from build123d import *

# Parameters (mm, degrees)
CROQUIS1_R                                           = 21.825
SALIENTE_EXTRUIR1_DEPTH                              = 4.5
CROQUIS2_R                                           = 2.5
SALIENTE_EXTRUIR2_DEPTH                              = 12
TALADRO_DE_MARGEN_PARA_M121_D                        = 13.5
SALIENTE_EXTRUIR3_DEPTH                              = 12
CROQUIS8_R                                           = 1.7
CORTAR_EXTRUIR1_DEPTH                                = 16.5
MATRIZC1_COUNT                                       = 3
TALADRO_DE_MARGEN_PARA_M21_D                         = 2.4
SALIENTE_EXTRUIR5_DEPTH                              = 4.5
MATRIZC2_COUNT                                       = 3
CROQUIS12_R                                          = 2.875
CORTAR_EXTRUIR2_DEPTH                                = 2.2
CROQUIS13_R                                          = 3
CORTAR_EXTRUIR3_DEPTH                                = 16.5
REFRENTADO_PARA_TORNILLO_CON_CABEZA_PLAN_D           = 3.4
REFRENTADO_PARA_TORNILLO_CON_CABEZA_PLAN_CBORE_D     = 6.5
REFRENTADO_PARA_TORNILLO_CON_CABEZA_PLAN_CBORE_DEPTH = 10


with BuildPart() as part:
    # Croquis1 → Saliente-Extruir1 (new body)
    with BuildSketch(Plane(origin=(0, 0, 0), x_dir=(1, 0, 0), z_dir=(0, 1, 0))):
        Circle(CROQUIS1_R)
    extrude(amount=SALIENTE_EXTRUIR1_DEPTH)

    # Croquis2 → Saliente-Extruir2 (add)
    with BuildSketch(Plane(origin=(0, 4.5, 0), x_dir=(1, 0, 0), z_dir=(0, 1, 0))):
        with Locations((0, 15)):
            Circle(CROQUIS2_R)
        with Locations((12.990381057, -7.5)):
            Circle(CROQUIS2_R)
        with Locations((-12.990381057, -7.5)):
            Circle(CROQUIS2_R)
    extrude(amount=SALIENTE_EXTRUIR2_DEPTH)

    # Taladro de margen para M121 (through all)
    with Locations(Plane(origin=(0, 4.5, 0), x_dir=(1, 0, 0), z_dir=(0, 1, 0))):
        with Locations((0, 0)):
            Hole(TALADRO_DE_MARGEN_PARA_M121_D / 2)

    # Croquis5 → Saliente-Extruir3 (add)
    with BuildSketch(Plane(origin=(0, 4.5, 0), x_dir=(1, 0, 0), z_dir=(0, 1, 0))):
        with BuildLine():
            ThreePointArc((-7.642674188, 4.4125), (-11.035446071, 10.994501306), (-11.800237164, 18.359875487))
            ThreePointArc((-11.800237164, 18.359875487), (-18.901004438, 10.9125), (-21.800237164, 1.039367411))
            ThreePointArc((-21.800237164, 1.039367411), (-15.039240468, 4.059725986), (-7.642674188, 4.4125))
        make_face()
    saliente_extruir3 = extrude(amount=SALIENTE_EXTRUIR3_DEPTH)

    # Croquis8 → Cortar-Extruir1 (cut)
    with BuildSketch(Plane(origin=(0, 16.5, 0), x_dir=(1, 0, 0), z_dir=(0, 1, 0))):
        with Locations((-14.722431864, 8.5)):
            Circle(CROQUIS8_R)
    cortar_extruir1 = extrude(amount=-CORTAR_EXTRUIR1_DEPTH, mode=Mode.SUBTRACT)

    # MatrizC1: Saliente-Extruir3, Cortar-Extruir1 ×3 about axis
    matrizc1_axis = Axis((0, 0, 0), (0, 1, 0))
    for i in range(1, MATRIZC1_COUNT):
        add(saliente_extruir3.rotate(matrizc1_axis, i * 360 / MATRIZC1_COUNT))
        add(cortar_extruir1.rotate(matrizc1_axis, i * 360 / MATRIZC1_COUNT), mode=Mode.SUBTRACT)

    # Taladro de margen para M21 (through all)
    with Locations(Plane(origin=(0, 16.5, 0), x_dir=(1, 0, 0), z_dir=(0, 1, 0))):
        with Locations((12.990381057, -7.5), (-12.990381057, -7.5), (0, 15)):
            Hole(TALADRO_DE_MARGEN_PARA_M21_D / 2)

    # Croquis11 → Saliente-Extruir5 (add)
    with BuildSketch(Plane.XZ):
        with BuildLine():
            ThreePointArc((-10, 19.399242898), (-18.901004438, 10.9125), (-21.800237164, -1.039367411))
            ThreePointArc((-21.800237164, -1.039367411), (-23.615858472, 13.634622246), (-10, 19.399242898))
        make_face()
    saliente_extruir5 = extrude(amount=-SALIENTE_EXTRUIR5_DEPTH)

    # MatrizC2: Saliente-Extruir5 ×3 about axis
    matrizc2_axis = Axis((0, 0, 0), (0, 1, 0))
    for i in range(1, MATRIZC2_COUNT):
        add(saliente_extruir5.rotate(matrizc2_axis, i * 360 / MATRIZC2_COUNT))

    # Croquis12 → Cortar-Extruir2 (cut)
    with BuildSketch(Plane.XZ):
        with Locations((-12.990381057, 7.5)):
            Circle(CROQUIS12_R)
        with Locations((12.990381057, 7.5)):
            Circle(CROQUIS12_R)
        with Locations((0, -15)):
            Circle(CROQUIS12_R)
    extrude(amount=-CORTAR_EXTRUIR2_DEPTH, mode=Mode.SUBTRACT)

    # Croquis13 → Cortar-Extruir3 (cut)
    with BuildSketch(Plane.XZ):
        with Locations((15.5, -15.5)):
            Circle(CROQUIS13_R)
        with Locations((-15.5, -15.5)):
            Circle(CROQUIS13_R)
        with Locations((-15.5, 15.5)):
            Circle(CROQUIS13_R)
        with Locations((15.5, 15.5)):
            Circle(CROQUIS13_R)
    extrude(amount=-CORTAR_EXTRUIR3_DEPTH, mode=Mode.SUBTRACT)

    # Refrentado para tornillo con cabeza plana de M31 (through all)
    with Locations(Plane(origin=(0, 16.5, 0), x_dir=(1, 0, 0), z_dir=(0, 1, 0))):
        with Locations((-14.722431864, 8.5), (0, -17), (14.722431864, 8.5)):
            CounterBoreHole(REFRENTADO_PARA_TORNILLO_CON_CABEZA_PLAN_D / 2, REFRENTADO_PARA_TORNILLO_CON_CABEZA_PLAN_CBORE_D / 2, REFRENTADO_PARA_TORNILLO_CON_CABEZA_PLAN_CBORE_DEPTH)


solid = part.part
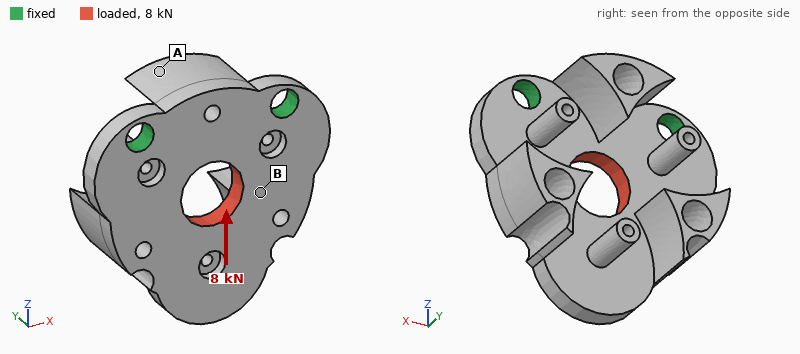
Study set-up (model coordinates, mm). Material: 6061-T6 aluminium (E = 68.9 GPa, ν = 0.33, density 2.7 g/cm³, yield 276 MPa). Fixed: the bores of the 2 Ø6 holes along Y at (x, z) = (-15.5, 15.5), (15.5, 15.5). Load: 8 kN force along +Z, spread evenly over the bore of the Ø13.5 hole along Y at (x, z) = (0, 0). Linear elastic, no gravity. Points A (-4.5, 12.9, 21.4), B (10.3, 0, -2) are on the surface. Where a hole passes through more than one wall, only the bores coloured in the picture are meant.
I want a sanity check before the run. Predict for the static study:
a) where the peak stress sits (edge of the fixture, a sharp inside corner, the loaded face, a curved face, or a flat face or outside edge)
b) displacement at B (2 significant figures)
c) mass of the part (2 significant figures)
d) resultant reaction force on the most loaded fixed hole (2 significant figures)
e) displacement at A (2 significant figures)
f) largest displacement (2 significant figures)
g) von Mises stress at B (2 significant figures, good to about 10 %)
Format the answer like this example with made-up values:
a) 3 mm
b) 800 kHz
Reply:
a) a curved face
b) 21 µm
c) 27 g
d) 4.2 kN
e) 15 µm
f) 44 µm
g) 40 MPa
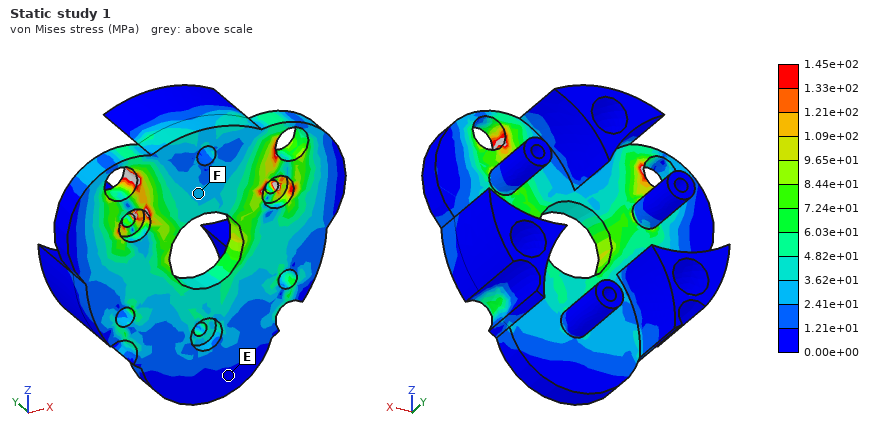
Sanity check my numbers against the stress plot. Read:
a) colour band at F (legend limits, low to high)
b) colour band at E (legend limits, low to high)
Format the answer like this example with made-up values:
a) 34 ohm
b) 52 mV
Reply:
a) 2.41e+01 to 3.62e+01 MPa
b) 0.00e+00 to 1.21e+01 MPa
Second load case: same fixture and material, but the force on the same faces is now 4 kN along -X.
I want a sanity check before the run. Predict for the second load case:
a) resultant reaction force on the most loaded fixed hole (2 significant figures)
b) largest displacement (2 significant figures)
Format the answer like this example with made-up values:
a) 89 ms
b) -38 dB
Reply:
a) 2.5 kN
b) 36 µm
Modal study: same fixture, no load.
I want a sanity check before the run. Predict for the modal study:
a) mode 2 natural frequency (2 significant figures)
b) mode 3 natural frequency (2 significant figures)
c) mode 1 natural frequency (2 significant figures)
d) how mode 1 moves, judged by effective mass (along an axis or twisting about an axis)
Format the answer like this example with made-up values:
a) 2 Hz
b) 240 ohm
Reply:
a) 5600 Hz
b) 10000 Hz
c) 2200 Hz
d) along Y
